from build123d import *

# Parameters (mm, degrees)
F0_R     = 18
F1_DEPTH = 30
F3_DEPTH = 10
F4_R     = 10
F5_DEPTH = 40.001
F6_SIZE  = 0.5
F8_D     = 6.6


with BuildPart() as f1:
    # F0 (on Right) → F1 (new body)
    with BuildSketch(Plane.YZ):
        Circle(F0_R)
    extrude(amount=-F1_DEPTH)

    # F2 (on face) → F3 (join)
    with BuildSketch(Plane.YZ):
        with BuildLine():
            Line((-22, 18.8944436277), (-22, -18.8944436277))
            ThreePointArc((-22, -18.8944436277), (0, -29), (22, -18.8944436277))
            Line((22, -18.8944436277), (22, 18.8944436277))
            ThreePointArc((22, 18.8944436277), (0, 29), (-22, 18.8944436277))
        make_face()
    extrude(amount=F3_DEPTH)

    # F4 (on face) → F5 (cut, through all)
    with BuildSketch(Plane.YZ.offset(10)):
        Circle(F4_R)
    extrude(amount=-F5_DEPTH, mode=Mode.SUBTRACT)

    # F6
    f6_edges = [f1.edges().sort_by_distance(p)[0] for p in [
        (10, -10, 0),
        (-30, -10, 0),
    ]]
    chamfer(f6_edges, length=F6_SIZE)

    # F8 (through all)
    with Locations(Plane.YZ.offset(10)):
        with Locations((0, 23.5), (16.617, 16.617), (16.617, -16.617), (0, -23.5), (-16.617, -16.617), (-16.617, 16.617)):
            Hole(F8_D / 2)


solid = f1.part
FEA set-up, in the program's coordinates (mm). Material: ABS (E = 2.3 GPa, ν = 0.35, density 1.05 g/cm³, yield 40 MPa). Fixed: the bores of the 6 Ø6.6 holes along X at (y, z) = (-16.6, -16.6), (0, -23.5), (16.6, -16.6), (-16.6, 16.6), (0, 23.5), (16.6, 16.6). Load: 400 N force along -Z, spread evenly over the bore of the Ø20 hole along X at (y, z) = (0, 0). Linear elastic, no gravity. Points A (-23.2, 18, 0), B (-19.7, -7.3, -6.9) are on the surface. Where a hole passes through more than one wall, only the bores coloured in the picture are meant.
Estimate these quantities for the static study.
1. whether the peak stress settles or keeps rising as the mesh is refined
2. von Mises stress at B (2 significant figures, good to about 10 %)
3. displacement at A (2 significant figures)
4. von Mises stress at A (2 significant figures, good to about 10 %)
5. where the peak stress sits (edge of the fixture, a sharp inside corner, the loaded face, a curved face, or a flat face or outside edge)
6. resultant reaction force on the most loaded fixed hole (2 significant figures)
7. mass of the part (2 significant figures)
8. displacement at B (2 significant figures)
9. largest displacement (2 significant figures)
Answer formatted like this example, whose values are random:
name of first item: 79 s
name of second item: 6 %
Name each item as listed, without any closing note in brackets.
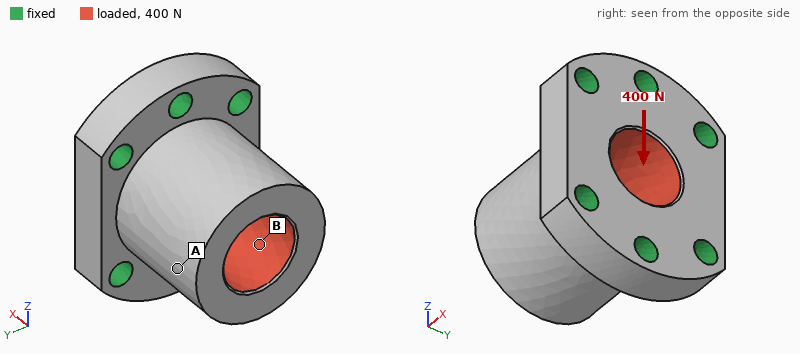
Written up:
whether the peak stress settles or keeps rising as the mesh is refined: keeps rising
von Mises stress at B: 0.60 MPa
displacement at A: 21 µm
von Mises stress at A: 0.24 MPa
where the peak stress sits: a sharp inside corner
resultant reaction force on the most loaded fixed hole: 110 N
mass of the part: 41 g
displacement at B: 20 µm
largest displacement: 29 µm
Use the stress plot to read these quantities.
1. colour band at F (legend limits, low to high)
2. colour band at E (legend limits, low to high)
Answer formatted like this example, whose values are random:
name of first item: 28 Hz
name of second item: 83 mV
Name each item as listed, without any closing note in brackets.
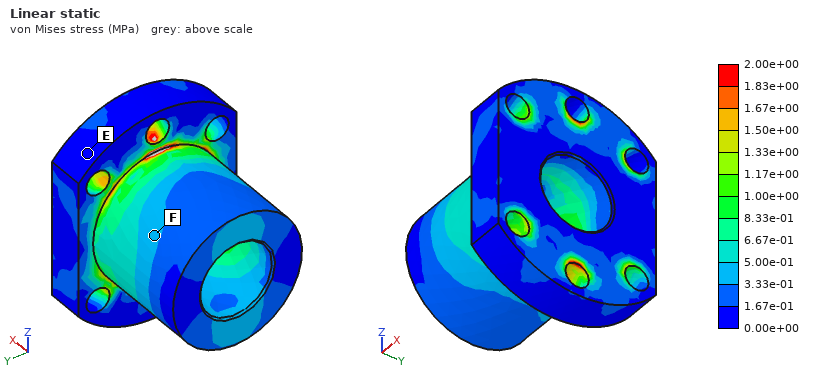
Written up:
colour band at F: 3.33e-01 to 5.00e-01 MPa
colour band at E: 0.00e+00 to 1.67e-01 MPa
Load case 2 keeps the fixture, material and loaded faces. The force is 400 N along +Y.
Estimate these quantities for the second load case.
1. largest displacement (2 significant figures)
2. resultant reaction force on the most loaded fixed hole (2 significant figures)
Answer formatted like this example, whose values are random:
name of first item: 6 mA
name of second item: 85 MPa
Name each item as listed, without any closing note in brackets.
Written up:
largest displacement: 38 µm
resultant reaction force on the most loaded fixed hole: 130 N
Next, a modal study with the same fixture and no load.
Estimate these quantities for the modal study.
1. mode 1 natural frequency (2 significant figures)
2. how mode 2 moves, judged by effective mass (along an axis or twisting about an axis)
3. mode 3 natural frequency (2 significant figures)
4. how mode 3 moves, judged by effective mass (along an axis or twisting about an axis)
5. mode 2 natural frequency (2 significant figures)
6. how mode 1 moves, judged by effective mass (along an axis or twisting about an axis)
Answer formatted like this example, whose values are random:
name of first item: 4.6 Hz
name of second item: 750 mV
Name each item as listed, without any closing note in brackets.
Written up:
mode 1 natural frequency: 3500 Hz
how mode 2 moves, judged by effective mass: along Z
mode 3 natural frequency: 6500 Hz
how mode 3 moves, judged by effective mass: twisting about X
mode 2 natural frequency: 4100 Hz
how mode 1 moves, judged by effective mass: along Y
